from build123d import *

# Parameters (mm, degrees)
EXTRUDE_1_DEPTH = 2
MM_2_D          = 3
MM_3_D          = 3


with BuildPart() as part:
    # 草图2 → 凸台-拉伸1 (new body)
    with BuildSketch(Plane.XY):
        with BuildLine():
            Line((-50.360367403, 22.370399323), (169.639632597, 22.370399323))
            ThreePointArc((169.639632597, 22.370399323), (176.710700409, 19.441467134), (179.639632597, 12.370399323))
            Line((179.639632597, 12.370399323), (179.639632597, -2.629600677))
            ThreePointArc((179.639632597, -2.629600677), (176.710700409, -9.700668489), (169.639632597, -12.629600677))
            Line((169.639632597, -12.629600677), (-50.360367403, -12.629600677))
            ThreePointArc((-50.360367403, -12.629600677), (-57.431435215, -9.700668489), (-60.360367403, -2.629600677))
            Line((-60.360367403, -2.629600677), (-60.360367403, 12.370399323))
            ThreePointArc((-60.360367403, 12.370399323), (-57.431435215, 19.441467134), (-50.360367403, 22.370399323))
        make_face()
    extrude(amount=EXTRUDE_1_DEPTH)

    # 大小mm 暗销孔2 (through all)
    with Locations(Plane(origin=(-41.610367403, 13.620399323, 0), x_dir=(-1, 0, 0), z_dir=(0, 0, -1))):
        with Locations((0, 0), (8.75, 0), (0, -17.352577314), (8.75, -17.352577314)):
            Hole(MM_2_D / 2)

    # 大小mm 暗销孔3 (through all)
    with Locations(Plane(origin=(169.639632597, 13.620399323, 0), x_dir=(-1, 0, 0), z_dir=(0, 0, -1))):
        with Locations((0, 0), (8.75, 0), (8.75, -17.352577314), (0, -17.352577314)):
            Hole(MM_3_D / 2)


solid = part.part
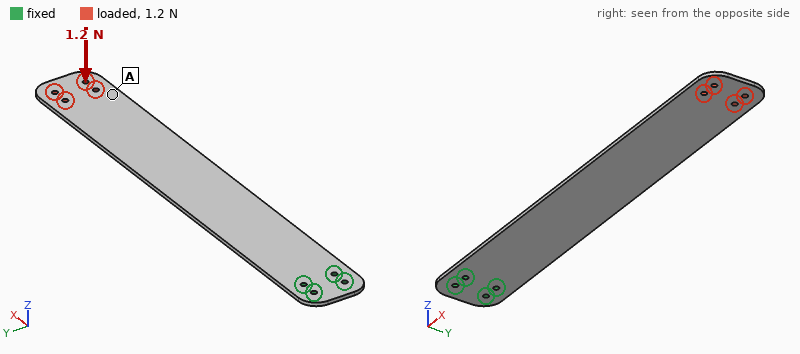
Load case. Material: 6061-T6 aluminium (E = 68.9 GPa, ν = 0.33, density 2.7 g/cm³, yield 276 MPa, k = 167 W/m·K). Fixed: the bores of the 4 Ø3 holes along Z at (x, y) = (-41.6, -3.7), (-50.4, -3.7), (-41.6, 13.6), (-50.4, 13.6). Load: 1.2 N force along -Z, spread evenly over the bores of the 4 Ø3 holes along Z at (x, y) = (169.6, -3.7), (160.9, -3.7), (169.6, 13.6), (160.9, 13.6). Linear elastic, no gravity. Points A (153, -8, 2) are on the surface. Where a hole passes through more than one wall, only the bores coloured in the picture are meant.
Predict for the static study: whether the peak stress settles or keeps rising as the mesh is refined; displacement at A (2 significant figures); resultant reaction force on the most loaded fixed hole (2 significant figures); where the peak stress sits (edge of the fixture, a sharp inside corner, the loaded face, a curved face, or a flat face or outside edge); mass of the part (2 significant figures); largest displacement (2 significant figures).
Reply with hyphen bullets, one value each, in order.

- keeps rising
- 2.0 mm
- 5.1 N
- edge of the fixture
- 45 g
- 2.4 mm
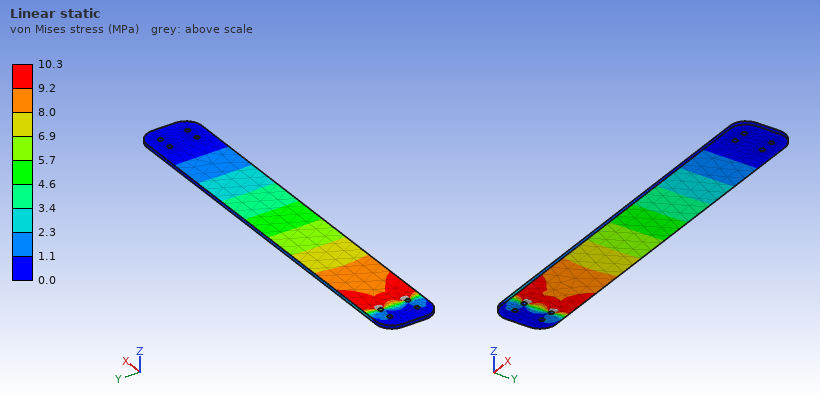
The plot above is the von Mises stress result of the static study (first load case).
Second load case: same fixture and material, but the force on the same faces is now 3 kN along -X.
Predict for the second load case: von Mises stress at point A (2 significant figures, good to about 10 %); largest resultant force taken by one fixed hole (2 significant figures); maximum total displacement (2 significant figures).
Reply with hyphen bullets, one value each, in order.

- 43 MPa
- 1.1 kN
- 0.13 mm
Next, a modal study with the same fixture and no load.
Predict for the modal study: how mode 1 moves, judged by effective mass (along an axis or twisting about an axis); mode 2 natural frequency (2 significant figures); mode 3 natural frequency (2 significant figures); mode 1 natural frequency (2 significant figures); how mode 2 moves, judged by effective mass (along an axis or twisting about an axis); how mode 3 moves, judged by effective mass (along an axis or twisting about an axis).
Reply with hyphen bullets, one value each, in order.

- along Z
- 210 Hz
- 420 Hz
- 34 Hz
- along Z
- twisting about X
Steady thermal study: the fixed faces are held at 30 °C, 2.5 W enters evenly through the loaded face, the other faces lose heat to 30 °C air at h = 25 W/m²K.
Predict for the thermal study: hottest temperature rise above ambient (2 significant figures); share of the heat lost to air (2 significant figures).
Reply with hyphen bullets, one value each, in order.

- 15 K
- 88 %
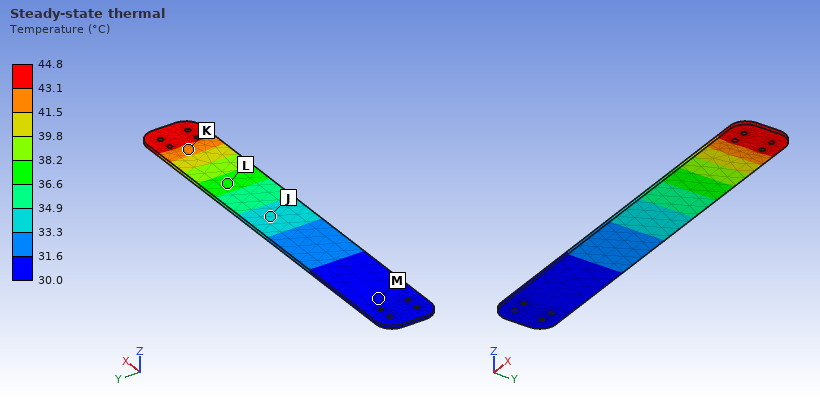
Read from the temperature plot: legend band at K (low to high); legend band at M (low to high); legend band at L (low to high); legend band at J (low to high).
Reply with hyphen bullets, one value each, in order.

- 41.5 to 43.1 °C
- 30.0 to 31.6 °C
- 36.6 to 38.2 °C
- 33.3 to 34.9 °C
